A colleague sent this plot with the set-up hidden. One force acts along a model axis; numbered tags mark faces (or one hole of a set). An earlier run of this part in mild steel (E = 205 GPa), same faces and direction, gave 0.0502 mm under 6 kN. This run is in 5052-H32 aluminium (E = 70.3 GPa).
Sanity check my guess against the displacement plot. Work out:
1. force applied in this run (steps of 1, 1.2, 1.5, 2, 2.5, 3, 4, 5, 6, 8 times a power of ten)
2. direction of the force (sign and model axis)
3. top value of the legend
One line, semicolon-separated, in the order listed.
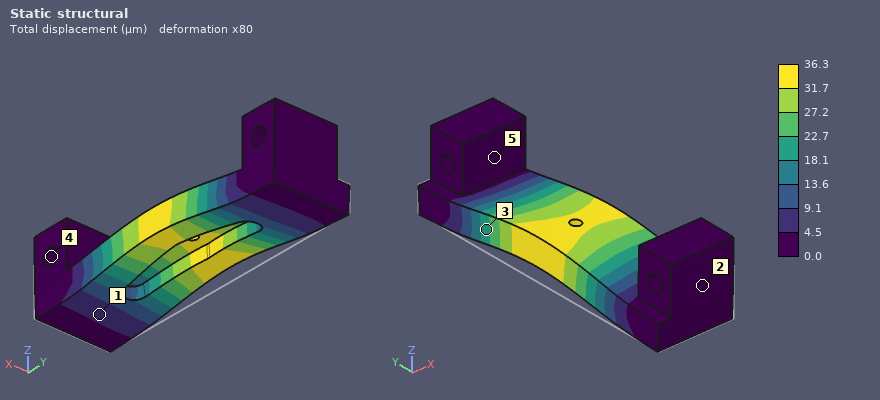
1.5 kN; +Z; 36.3 µm
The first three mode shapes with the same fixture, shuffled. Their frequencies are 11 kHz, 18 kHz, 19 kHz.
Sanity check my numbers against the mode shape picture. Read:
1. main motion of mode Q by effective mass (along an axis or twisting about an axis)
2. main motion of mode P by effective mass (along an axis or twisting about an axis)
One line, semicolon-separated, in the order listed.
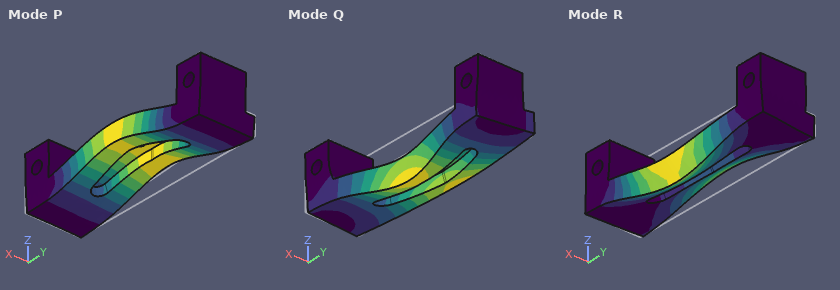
along X; along Z
